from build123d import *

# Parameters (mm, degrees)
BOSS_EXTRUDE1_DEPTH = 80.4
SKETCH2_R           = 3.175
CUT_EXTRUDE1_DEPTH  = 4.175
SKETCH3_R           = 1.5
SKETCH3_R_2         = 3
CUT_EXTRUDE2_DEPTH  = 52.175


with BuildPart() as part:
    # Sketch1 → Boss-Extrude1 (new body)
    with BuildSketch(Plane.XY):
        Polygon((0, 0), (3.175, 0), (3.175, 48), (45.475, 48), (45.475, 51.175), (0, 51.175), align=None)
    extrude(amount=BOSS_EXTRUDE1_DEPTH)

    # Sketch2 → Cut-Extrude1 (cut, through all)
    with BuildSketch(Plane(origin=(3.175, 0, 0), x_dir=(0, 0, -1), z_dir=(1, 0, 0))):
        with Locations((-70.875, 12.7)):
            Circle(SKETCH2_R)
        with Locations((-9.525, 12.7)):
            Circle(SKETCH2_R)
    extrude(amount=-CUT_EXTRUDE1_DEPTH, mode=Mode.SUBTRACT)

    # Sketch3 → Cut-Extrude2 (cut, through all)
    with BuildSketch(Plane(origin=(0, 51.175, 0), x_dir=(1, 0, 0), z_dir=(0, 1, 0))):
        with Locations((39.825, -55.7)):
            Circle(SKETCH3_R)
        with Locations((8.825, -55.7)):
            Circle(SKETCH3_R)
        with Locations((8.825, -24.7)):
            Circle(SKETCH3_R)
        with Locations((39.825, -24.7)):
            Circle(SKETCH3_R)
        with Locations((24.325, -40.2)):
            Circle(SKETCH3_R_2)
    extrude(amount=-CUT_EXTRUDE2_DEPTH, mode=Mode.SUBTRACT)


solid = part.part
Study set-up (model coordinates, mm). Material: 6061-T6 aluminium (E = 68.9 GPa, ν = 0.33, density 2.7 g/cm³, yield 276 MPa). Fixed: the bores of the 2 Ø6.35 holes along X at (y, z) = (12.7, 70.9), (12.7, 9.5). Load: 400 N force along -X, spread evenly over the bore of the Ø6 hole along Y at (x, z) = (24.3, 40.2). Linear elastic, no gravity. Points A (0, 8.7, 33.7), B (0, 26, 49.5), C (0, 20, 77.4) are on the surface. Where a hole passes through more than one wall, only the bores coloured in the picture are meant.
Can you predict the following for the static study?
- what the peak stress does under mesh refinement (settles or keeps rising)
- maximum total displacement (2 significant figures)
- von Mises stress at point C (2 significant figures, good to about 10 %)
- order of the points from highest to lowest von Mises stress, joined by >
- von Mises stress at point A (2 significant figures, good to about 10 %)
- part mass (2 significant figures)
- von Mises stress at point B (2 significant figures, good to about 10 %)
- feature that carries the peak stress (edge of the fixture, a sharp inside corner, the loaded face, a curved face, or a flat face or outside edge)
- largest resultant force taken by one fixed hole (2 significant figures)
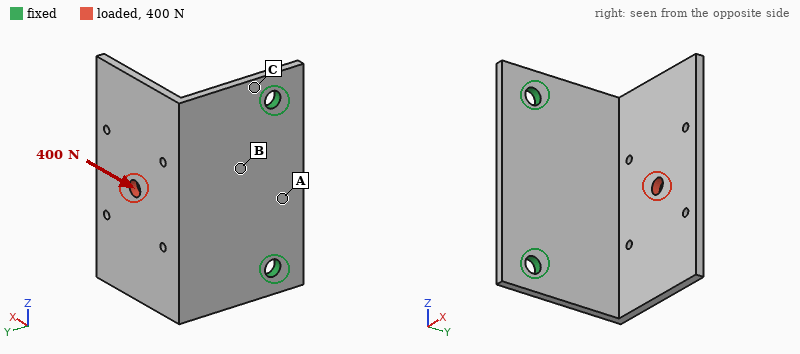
keeps rising
1.0 mm
110 MPa
C > B > A
23 MPa
63 g
48 MPa
edge of the fixture
200 N
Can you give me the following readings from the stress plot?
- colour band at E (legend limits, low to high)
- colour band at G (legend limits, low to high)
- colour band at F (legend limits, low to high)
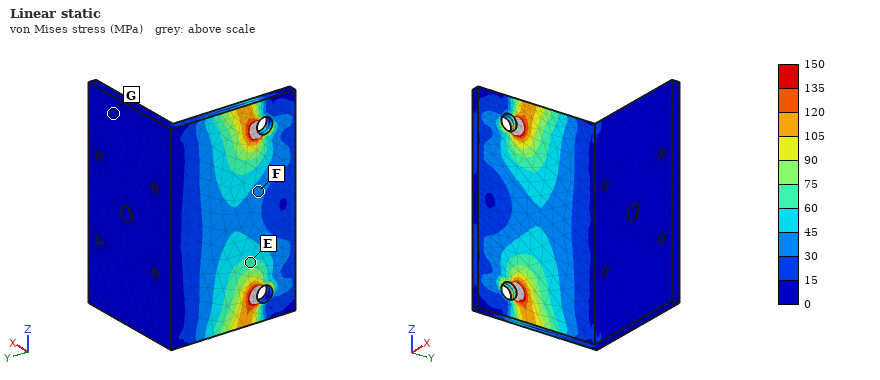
60 to 75 MPa
0 to 15 MPa
30 to 45 MPa
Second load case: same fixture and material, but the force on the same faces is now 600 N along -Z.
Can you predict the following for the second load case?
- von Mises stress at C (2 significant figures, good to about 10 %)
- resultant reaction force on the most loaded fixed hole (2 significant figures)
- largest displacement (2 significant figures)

74 MPa
510 N
0.50 mm
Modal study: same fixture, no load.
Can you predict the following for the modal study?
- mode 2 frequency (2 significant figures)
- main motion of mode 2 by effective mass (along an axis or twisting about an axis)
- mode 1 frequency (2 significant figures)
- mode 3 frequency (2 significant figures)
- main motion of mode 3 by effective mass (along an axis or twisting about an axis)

1000 Hz
along Z
530 Hz
1400 Hz
along X
